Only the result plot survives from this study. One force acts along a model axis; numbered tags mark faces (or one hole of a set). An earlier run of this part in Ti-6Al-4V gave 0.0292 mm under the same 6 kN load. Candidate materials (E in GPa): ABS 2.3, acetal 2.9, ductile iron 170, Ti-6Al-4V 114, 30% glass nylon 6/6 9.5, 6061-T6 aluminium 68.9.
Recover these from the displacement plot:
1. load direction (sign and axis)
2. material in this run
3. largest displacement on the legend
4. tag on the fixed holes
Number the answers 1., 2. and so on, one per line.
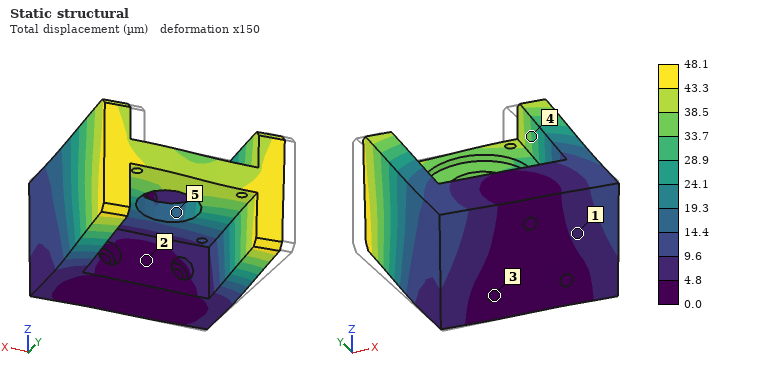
1. +X
2. 6061-T6 aluminium
3. 48.1 µm
4. 3
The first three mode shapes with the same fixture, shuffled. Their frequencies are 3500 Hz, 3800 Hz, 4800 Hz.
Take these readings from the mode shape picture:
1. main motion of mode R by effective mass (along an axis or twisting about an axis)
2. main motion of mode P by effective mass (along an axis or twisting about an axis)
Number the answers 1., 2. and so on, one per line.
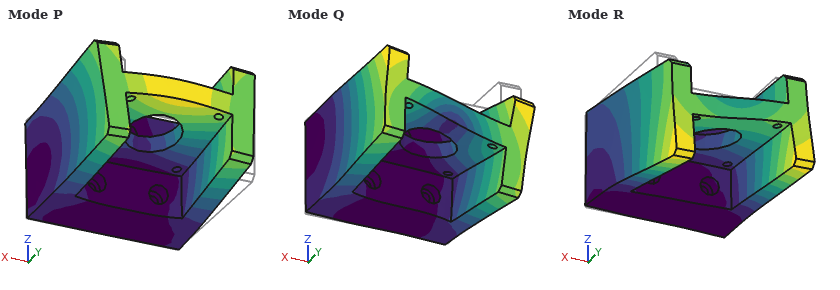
1. along X
2. along Z
